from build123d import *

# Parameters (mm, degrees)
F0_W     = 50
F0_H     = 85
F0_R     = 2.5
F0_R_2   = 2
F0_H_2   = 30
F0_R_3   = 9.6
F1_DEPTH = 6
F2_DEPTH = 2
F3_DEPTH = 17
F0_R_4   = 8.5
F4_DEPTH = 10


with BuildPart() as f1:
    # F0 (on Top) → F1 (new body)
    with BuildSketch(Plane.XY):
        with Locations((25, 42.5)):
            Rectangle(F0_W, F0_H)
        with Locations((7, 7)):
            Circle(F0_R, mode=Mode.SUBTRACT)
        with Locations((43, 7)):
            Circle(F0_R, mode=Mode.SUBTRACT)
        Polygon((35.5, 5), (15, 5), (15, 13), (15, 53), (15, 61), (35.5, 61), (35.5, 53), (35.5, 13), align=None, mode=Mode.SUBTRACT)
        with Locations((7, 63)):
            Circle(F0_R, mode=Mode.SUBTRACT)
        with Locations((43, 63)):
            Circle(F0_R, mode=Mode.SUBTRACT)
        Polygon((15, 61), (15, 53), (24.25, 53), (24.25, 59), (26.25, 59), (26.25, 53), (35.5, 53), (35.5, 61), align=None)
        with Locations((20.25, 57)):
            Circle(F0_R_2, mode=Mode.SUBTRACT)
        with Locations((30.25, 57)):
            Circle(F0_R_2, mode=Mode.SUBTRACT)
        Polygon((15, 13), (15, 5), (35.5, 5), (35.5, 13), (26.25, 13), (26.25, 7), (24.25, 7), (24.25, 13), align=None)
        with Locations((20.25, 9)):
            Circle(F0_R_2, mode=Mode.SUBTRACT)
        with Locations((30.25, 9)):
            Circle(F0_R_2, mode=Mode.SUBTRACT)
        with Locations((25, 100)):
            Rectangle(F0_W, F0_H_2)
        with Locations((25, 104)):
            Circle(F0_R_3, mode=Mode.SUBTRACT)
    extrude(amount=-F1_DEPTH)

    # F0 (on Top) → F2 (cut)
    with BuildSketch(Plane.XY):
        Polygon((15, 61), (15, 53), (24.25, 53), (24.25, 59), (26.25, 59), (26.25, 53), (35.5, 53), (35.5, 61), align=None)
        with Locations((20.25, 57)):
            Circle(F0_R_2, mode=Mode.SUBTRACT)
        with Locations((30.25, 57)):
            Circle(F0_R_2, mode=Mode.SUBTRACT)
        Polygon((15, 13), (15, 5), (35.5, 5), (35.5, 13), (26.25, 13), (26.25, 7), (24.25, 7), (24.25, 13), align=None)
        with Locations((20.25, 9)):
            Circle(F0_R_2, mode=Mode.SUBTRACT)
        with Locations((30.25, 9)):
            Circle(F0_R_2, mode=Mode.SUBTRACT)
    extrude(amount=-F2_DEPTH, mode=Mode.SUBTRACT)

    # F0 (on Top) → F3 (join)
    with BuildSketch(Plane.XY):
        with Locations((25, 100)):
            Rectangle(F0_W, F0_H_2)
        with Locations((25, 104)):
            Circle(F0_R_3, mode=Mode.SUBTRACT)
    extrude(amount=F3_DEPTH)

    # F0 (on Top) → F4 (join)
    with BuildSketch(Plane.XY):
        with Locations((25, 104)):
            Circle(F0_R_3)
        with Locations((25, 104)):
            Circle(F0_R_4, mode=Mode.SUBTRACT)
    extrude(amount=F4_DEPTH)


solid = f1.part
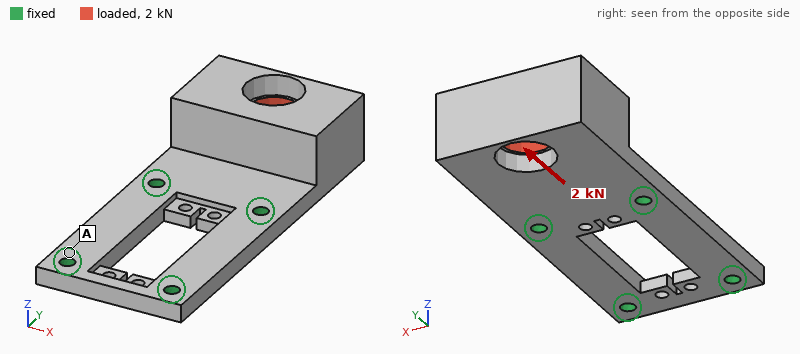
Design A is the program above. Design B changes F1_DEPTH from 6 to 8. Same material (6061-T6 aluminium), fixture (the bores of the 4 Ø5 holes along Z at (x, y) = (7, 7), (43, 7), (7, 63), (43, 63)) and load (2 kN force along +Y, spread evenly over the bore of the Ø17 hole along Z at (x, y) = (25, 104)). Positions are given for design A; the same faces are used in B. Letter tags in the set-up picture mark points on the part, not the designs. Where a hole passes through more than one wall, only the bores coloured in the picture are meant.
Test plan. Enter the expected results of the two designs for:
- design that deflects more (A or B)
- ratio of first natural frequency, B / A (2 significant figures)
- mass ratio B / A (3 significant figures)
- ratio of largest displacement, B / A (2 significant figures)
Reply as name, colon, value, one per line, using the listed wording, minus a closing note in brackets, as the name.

design that deflects more: A
ratio of first natural frequency, B / A: 1.4
mass ratio B / A: 1.19
ratio of largest displacement, B / A: 0.51
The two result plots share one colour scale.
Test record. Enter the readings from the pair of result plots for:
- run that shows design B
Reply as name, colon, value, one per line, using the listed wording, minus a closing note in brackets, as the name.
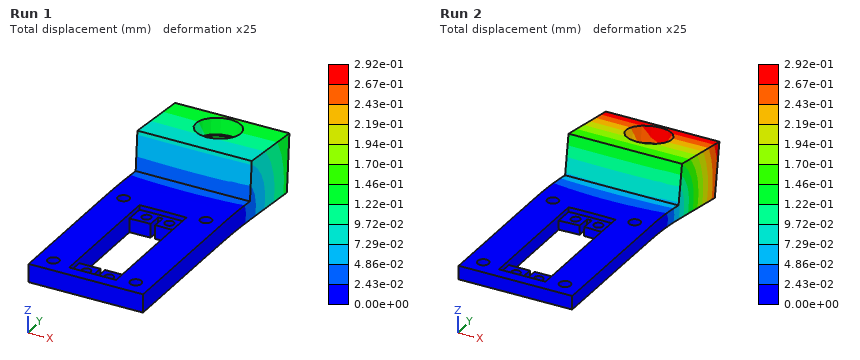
run that shows design B: Run 1
